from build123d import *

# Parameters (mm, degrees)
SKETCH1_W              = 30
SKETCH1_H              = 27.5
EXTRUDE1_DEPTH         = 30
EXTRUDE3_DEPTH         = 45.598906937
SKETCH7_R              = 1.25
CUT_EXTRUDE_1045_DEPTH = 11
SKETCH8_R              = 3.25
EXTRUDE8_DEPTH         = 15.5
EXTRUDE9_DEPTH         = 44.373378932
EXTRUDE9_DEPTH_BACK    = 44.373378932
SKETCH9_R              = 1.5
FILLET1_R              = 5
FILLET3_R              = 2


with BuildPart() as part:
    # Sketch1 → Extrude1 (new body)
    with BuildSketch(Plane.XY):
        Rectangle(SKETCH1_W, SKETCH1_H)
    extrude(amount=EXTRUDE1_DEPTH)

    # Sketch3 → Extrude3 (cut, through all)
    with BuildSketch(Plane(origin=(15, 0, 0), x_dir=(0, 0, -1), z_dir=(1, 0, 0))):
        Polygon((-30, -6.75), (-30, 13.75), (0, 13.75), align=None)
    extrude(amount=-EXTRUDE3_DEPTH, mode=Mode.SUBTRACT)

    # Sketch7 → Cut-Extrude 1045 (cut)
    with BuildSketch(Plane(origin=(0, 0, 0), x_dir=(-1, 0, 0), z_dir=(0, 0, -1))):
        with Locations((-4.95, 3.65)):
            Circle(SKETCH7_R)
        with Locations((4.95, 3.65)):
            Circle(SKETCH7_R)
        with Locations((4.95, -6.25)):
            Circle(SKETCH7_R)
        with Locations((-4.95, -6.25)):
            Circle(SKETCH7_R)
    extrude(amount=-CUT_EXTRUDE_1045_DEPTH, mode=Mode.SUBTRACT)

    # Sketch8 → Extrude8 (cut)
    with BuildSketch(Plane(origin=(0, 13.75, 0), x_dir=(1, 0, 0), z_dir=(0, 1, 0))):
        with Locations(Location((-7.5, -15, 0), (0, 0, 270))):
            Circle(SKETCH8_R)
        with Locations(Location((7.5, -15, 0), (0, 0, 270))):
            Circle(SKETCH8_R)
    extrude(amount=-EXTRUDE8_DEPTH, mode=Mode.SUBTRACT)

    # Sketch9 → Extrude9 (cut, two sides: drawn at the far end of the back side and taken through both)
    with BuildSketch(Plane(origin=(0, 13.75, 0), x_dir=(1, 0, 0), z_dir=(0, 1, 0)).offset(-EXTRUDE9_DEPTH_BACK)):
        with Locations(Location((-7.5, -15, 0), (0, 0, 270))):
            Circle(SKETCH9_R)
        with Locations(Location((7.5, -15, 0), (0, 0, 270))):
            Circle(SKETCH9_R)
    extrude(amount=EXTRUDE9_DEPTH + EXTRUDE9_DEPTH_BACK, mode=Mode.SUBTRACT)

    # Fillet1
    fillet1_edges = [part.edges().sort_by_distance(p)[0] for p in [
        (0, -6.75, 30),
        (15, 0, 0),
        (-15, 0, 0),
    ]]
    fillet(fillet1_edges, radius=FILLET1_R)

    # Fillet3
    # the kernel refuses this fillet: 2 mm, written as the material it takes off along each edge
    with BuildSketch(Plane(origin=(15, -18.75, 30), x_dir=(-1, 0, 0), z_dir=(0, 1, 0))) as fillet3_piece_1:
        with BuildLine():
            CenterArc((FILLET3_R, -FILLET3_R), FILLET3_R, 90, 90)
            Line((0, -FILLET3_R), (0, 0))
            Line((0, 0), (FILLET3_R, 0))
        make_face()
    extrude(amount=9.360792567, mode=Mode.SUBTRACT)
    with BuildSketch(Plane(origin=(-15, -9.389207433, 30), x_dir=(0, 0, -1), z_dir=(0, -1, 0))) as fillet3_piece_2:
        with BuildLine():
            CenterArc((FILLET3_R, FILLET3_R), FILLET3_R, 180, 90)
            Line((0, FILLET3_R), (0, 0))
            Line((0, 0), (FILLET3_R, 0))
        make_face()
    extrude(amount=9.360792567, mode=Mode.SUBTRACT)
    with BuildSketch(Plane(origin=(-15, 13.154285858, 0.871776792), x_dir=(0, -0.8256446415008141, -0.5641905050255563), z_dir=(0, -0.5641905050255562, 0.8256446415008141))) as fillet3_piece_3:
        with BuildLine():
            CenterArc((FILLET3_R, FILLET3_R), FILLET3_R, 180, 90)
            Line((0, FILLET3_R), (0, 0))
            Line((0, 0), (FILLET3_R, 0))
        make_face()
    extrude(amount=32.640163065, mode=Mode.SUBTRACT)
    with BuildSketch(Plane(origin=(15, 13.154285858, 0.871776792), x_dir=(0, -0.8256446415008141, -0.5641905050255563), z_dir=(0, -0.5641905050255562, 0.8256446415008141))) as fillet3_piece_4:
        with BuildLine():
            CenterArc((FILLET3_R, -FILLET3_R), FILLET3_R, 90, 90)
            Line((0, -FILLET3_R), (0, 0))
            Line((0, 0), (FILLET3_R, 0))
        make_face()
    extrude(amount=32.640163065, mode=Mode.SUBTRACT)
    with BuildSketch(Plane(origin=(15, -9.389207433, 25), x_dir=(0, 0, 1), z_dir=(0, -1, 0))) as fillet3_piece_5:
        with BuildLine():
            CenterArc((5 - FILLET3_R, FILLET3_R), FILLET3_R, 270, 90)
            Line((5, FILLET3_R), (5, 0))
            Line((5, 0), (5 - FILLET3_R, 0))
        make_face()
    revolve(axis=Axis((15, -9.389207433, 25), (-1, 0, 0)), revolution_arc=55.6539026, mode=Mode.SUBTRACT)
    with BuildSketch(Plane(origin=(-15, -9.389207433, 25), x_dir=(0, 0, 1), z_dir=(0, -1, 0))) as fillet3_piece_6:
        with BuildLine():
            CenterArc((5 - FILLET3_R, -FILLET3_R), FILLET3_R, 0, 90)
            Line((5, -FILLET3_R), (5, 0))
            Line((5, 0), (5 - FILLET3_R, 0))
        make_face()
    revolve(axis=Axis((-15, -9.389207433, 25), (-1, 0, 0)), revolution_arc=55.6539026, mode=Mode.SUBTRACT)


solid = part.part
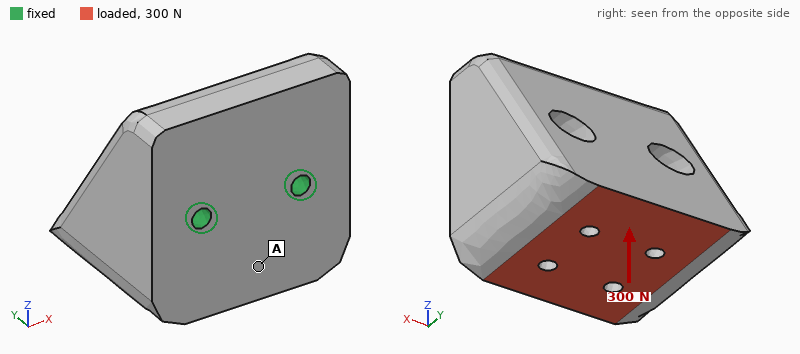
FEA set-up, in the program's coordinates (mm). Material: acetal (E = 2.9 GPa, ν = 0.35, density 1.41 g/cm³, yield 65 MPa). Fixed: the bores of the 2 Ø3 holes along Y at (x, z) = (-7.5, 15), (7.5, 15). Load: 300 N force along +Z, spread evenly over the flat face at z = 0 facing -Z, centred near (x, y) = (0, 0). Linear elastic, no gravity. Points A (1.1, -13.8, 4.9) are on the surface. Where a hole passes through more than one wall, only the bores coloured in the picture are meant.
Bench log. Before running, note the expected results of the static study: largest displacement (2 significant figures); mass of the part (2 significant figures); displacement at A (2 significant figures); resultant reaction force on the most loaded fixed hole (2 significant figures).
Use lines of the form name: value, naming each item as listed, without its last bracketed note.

largest displacement: 53 µm
mass of the part: 20 g
displacement at A: 10 µm
resultant reaction force on the most loaded fixed hole: 150 N
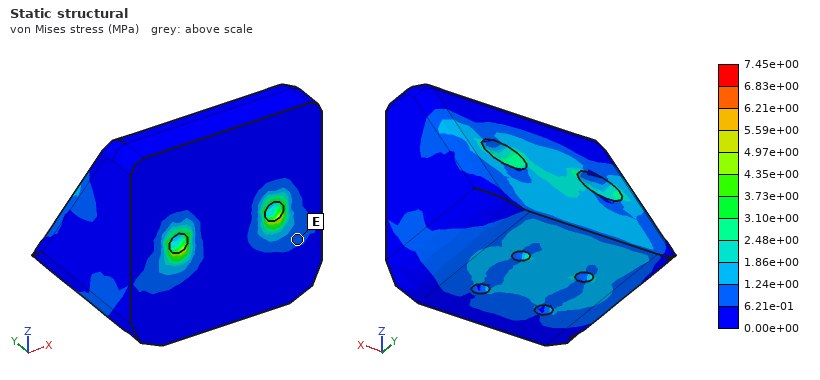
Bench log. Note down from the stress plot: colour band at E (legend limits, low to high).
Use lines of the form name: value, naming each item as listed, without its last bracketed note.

colour band at E: 6.21e-01 to 1.24e+00 MPa
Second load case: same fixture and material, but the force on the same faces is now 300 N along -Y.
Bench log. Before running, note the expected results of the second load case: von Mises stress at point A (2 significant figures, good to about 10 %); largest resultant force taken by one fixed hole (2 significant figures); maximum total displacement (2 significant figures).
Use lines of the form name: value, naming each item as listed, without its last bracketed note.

von Mises stress at point A: 1.3 MPa
largest resultant force taken by one fixed hole: 150 N
maximum total displacement: 85 µm
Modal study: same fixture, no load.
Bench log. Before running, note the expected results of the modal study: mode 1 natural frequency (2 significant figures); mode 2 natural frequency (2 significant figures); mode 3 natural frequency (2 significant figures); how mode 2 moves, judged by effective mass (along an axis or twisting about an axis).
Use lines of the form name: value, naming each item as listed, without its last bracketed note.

mode 1 natural frequency: 4600 Hz
mode 2 natural frequency: 6600 Hz
mode 3 natural frequency: 8000 Hz
how mode 2 moves, judged by effective mass: along X
